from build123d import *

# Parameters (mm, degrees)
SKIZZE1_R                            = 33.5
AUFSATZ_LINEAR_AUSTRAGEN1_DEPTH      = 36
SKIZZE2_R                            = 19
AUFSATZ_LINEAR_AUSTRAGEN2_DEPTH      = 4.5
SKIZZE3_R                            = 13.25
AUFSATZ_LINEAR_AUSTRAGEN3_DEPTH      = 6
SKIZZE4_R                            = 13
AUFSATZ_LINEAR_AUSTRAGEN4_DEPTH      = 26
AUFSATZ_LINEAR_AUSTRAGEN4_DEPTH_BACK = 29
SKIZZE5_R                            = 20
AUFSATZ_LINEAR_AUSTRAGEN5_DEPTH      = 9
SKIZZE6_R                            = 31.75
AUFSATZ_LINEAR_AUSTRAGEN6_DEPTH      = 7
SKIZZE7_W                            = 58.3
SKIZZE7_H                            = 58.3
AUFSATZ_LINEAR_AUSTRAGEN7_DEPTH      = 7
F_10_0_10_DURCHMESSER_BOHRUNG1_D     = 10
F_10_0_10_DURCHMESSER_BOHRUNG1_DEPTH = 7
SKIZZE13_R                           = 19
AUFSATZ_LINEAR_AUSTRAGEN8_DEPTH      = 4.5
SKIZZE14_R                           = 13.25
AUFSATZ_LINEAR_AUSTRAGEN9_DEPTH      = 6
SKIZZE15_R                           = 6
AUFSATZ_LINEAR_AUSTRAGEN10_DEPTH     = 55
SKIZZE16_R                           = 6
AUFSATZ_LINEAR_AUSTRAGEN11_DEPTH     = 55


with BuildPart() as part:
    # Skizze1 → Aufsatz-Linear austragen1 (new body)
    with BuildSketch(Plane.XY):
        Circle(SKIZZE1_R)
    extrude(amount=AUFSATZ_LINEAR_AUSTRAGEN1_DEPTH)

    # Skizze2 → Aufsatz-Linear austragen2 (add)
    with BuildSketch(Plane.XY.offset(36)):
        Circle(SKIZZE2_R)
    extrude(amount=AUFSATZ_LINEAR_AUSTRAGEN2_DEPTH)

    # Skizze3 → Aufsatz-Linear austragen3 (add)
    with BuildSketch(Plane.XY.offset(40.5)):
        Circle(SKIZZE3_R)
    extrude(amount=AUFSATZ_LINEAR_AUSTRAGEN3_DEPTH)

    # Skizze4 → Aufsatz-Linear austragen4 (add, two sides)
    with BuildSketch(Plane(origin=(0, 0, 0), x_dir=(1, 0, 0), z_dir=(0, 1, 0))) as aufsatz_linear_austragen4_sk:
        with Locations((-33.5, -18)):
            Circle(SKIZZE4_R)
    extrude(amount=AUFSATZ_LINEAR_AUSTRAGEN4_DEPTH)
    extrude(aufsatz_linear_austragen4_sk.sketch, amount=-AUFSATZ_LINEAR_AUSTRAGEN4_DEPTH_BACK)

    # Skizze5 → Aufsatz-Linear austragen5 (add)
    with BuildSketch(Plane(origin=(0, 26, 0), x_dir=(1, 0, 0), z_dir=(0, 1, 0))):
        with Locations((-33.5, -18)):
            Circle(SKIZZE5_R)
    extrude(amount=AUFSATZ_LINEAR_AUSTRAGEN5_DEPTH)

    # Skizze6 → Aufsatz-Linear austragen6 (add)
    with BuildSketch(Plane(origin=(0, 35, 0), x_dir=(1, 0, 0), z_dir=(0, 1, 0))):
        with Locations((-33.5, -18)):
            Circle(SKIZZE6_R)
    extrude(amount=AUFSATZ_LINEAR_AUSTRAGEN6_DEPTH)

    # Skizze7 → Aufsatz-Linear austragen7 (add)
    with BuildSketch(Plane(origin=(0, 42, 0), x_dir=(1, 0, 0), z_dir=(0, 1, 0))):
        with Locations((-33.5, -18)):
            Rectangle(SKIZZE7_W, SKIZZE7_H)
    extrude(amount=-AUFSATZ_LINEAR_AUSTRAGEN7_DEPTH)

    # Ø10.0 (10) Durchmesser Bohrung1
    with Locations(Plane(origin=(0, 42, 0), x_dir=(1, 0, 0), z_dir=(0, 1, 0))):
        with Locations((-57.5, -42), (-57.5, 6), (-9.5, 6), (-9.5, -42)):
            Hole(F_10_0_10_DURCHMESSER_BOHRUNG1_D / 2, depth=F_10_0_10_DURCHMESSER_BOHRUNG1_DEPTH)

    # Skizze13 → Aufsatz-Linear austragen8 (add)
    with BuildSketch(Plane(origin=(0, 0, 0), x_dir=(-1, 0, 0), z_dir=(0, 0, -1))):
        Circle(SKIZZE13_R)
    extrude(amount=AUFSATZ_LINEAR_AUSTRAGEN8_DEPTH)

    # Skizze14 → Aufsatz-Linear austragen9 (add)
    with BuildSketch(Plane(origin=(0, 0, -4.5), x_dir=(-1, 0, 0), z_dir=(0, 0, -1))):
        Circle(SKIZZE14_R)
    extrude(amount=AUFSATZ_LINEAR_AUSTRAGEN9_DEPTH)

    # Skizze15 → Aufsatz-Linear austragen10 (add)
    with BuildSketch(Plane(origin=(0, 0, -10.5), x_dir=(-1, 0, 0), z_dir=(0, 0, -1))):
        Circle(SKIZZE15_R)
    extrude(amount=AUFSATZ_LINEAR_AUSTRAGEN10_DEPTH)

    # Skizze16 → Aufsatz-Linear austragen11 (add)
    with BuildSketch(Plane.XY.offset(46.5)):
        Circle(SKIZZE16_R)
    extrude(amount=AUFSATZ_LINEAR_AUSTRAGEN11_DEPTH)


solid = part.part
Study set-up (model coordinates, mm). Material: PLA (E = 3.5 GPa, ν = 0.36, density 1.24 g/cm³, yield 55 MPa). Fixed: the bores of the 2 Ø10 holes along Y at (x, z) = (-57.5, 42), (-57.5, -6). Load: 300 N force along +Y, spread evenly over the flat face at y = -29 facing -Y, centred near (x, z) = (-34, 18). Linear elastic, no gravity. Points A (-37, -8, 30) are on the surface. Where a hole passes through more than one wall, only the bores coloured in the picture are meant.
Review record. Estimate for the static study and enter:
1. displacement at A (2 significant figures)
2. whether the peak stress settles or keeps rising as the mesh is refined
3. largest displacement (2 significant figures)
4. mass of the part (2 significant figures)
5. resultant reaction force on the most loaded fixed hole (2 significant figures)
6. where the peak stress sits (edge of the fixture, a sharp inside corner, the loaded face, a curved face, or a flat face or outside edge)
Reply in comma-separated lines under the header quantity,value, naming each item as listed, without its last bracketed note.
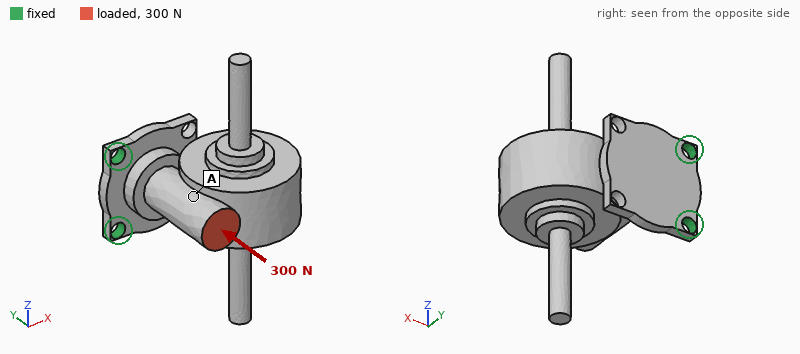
quantity,value
displacement at A,0.50 mm
whether the peak stress settles or keeps rising as the mesh is refined,keeps rising
largest displacement,1.0 mm
mass of the part,260 g
resultant reaction force on the most loaded fixed hole,150 N
where the peak stress sits,edge of the fixture
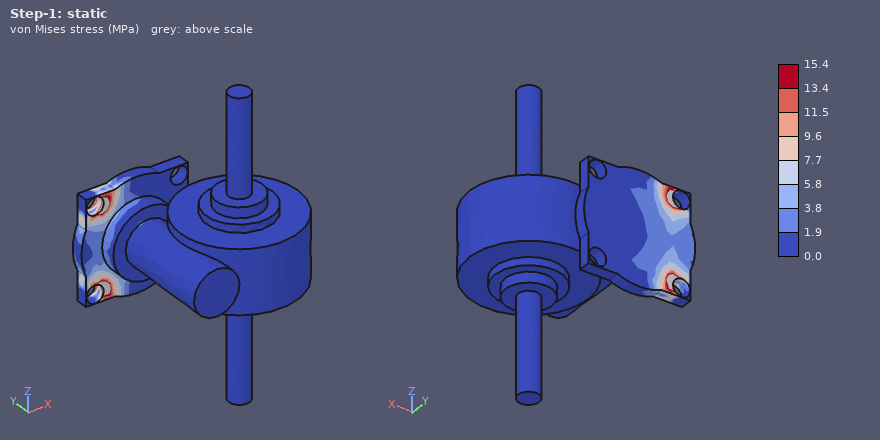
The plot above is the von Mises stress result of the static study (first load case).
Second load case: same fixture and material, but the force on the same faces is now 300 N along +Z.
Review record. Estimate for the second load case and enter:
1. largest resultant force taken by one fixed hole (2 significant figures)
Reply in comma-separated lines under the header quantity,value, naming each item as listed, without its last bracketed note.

quantity,value
largest resultant force taken by one fixed hole,540 N
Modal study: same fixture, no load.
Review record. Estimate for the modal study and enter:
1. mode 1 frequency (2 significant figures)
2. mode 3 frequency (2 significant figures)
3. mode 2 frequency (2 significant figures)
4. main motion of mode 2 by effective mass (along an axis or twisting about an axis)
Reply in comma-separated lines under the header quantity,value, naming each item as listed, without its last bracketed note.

quantity,value
mode 1 frequency,110 Hz
mode 3 frequency,660 Hz
mode 2 frequency,340 Hz
main motion of mode 2 by effective mass,along Z
